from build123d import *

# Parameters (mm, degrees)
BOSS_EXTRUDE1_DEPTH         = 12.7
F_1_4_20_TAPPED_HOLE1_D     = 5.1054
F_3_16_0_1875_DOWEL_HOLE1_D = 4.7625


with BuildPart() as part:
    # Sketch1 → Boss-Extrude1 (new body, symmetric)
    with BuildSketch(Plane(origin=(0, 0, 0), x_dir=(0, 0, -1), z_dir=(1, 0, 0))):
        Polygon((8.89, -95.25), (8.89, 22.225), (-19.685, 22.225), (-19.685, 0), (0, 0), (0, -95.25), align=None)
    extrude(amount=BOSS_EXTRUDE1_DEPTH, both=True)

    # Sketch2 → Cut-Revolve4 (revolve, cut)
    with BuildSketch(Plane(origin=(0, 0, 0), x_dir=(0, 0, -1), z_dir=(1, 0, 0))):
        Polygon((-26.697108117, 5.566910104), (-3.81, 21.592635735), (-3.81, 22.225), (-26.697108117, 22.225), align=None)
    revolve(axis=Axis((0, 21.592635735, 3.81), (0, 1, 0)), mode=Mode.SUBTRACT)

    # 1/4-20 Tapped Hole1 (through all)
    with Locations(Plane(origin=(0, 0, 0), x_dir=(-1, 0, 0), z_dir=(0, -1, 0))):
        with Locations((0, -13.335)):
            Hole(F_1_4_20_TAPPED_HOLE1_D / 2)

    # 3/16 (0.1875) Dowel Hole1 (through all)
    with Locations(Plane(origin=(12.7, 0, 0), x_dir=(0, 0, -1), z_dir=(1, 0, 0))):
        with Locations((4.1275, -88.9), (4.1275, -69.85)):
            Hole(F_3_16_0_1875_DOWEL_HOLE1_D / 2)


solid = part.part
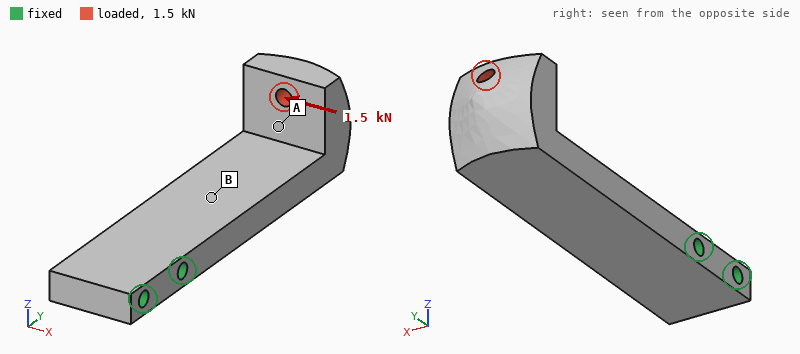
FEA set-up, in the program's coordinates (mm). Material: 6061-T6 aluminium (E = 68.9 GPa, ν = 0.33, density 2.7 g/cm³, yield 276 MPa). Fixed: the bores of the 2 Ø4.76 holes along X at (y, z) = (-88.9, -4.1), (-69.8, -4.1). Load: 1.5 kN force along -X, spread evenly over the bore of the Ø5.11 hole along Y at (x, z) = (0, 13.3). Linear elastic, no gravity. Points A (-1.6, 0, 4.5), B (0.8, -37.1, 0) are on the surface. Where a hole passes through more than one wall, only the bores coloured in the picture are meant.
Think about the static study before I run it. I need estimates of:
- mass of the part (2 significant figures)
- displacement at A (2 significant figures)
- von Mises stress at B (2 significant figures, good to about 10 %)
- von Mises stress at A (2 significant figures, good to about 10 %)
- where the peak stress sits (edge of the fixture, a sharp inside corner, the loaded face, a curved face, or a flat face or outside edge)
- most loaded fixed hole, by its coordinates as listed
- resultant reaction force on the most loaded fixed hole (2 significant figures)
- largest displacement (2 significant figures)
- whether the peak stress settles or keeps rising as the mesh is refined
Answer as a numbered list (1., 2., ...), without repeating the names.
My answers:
1. 83 g
2. 0.37 mm
3. 100 MPa
4. 22 MPa
5. edge of the fixture
6. (-69.8, -4.1)
7. 1.6 kN
8. 0.66 mm
9. keeps rising
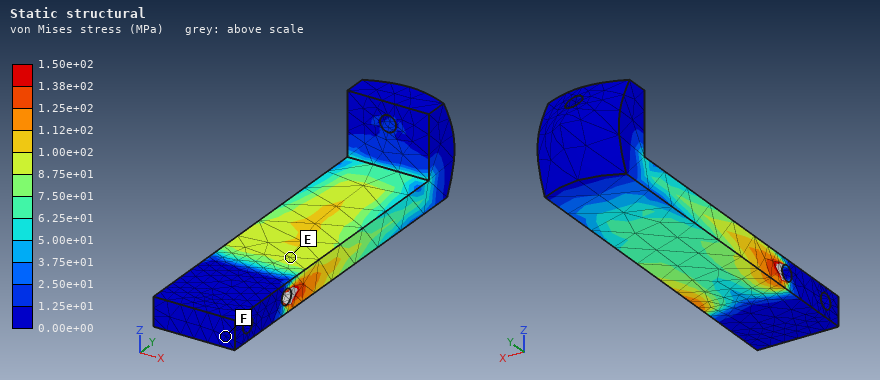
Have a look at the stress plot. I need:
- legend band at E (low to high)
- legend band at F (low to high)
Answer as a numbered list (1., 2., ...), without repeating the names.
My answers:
1. 8.75e+01 to 1.00e+02 MPa
2. 0.00e+00 to 1.25e+01 MPa
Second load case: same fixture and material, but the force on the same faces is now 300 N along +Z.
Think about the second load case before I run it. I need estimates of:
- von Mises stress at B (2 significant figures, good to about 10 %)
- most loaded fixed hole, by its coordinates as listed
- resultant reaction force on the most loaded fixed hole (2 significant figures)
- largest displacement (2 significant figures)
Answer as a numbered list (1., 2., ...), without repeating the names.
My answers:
1. 40 MPa
2. (-69.8, -4.1)
3. 500 N
4. 0.58 mm
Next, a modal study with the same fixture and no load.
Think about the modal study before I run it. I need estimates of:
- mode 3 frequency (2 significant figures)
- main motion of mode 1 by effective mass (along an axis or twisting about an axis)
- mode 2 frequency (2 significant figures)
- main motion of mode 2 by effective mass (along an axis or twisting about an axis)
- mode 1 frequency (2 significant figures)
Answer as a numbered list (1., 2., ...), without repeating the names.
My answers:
1. 3600 Hz
2. along Z
3. 1800 Hz
4. along X
5. 680 Hz
